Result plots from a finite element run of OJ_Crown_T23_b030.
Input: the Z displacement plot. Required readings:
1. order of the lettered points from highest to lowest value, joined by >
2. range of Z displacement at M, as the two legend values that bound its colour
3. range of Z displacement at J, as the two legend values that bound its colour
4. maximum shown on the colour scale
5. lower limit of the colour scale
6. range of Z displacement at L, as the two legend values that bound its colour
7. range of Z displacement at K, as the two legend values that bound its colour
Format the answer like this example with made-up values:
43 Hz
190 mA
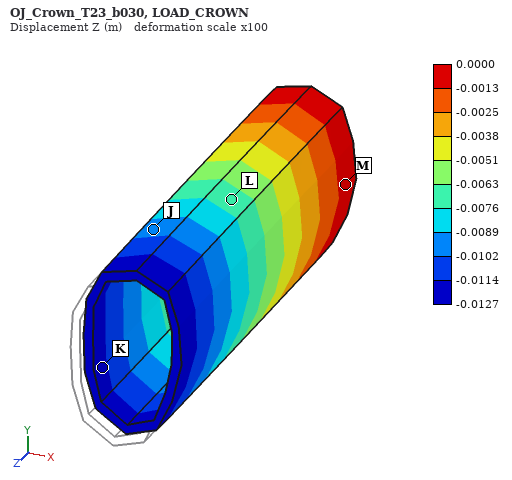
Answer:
M > L > J > K
-0.0013 to 0.0000 m
-0.0102 to -0.0089 m
0.0000 m
-0.0127 m
-0.0076 to -0.0063 m
-0.0127 to -0.0114 m
